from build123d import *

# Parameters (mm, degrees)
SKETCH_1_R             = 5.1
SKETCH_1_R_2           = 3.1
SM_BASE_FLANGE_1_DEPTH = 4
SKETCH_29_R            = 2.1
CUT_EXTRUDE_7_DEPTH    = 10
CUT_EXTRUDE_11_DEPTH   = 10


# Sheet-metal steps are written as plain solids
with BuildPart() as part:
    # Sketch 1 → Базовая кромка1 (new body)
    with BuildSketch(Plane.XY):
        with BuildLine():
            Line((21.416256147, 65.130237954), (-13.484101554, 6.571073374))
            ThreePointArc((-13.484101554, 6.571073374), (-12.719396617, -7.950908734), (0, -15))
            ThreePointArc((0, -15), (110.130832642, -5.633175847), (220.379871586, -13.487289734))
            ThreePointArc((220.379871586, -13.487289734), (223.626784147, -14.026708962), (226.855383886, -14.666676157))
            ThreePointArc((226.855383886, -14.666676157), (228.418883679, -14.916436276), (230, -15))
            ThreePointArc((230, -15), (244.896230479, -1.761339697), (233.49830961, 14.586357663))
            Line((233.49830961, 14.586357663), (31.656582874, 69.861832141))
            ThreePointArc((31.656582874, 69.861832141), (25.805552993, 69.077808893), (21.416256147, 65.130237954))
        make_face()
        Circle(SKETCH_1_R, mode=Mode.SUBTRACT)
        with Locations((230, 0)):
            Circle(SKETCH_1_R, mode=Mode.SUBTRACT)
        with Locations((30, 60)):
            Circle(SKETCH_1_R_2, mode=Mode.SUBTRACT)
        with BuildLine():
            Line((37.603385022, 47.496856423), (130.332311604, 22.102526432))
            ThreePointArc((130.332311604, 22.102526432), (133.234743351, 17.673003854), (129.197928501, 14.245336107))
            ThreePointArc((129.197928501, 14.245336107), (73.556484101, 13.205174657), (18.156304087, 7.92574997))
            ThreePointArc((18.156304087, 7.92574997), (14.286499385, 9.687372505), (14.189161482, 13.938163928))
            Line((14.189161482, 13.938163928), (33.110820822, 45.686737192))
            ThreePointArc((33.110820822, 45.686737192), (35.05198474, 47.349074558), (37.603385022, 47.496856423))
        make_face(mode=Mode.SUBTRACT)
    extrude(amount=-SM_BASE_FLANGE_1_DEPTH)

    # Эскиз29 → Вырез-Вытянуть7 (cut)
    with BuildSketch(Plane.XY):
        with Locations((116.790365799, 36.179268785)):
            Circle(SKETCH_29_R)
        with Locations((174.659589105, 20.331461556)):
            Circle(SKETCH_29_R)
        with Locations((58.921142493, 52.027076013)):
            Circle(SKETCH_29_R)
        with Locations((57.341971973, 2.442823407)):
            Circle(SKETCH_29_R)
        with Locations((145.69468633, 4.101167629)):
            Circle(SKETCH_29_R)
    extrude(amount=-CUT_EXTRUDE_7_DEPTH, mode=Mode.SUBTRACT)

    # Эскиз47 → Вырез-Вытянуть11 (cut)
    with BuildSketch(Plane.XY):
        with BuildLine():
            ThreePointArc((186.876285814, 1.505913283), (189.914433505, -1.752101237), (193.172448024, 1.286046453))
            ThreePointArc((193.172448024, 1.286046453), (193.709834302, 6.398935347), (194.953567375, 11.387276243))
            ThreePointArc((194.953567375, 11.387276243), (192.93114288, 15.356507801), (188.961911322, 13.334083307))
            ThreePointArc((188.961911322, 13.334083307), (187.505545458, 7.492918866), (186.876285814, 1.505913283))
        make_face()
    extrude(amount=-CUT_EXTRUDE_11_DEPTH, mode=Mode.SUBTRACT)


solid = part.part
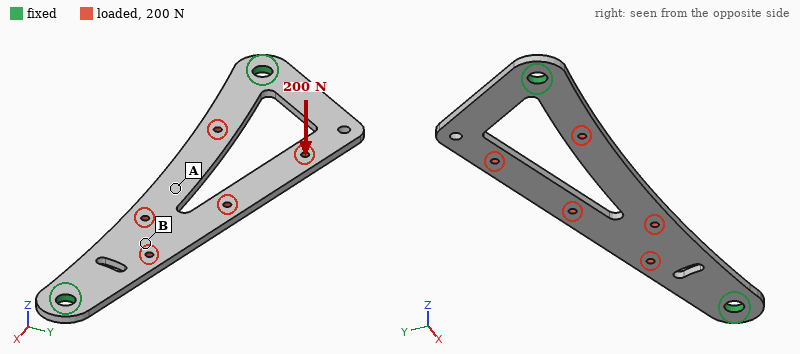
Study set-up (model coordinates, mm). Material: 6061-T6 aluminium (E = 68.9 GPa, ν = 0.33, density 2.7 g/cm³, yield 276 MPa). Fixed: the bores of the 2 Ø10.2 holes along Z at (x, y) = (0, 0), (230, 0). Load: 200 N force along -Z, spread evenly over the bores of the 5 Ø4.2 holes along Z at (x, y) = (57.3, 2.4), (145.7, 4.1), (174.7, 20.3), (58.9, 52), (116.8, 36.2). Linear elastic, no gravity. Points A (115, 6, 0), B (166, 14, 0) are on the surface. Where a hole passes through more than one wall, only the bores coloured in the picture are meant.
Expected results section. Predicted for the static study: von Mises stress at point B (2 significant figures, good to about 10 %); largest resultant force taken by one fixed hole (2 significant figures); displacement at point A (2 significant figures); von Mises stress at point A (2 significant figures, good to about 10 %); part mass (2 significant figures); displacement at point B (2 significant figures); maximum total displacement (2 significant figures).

13 MPa
110 N
0.58 mm
25 MPa
110 g
0.42 mm
0.87 mm
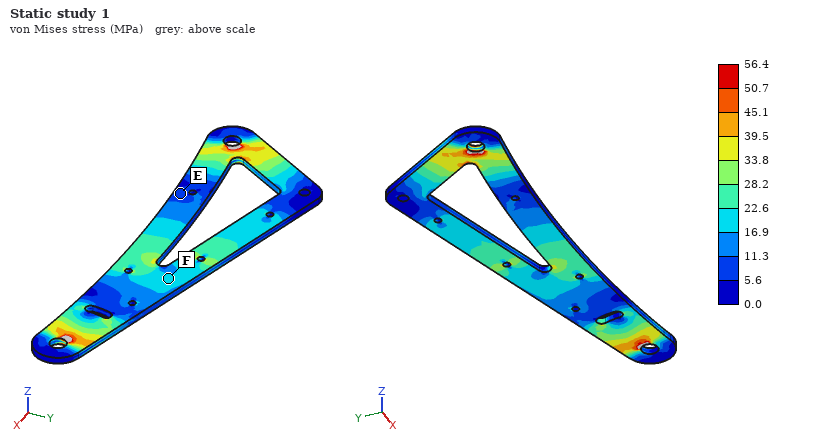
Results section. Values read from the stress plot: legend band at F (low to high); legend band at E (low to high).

16.9 to 22.6 MPa
5.6 to 11.3 MPa
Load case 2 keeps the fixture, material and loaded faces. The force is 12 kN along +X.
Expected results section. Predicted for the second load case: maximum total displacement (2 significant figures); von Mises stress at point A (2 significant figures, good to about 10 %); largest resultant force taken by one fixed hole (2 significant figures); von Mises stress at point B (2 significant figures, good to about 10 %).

0.20 mm
36 MPa
6.4 kN
24 MPa
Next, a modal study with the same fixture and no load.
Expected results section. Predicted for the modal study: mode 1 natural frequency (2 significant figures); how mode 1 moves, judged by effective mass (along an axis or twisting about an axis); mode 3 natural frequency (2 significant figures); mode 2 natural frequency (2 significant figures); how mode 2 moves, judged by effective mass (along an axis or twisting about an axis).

340 Hz
along Z
1000 Hz
590 Hz
twisting about X
